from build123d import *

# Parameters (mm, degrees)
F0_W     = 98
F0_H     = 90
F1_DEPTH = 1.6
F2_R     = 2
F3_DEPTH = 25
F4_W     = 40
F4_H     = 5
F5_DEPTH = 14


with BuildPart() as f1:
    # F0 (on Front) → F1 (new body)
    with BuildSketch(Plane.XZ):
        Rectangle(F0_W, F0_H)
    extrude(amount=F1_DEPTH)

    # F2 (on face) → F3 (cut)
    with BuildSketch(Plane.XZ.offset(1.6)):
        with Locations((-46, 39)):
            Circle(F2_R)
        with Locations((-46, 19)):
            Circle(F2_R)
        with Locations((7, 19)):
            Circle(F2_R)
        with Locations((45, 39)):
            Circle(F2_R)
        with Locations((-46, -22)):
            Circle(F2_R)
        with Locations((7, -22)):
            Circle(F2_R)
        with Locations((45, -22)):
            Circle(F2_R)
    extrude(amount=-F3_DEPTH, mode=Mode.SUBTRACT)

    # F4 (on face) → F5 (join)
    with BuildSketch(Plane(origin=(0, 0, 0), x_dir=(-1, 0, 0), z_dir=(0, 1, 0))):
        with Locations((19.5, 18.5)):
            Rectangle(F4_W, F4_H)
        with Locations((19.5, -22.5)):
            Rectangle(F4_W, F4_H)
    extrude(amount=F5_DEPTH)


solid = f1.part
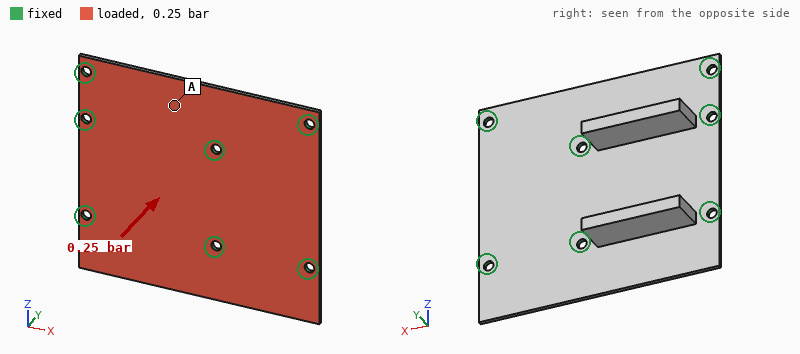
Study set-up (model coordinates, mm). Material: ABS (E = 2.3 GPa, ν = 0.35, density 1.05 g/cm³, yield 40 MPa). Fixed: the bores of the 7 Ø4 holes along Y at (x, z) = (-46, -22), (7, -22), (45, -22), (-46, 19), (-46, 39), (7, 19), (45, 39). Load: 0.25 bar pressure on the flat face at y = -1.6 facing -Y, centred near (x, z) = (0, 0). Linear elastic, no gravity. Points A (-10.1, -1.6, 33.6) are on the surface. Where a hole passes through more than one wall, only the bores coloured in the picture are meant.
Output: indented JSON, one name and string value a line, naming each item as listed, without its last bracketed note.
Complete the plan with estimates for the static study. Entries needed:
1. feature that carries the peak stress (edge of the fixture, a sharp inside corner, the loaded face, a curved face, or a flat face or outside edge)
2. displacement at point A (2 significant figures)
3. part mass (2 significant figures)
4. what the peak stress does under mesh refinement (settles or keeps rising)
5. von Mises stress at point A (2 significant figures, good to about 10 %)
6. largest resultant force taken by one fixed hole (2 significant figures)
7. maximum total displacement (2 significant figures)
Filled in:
{
  "feature that carries the peak stress": "edge of the fixture",
  "displacement at point A": "0.48 mm",
  "part mass": "21 g",
  "what the peak stress does under mesh refinement": "keeps rising",
  "von Mises stress at point A": "2.2 MPa",
  "largest resultant force taken by one fixed hole": "55 N",
  "maximum total displacement": "1.2 mm"
}
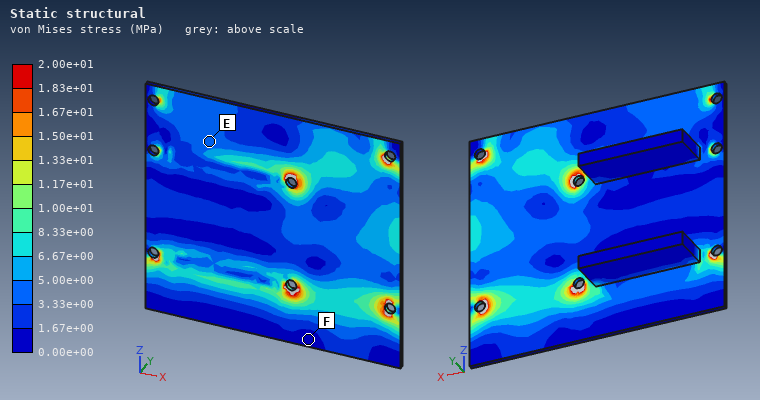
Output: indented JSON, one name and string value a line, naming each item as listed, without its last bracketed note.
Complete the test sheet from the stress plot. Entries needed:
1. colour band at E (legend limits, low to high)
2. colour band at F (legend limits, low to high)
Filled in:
{
  "colour band at E": "3.33e+00 to 5.00e+00 MPa",
  "colour band at F": "0.00e+00 to 1.67e+00 MPa"
}
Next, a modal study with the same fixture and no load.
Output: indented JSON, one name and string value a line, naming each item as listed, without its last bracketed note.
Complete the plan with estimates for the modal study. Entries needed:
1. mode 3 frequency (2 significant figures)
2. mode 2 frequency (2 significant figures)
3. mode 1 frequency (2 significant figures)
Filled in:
{
  "mode 3 frequency": "730 Hz",
  "mode 2 frequency": "720 Hz",
  "mode 1 frequency": "620 Hz"
}
